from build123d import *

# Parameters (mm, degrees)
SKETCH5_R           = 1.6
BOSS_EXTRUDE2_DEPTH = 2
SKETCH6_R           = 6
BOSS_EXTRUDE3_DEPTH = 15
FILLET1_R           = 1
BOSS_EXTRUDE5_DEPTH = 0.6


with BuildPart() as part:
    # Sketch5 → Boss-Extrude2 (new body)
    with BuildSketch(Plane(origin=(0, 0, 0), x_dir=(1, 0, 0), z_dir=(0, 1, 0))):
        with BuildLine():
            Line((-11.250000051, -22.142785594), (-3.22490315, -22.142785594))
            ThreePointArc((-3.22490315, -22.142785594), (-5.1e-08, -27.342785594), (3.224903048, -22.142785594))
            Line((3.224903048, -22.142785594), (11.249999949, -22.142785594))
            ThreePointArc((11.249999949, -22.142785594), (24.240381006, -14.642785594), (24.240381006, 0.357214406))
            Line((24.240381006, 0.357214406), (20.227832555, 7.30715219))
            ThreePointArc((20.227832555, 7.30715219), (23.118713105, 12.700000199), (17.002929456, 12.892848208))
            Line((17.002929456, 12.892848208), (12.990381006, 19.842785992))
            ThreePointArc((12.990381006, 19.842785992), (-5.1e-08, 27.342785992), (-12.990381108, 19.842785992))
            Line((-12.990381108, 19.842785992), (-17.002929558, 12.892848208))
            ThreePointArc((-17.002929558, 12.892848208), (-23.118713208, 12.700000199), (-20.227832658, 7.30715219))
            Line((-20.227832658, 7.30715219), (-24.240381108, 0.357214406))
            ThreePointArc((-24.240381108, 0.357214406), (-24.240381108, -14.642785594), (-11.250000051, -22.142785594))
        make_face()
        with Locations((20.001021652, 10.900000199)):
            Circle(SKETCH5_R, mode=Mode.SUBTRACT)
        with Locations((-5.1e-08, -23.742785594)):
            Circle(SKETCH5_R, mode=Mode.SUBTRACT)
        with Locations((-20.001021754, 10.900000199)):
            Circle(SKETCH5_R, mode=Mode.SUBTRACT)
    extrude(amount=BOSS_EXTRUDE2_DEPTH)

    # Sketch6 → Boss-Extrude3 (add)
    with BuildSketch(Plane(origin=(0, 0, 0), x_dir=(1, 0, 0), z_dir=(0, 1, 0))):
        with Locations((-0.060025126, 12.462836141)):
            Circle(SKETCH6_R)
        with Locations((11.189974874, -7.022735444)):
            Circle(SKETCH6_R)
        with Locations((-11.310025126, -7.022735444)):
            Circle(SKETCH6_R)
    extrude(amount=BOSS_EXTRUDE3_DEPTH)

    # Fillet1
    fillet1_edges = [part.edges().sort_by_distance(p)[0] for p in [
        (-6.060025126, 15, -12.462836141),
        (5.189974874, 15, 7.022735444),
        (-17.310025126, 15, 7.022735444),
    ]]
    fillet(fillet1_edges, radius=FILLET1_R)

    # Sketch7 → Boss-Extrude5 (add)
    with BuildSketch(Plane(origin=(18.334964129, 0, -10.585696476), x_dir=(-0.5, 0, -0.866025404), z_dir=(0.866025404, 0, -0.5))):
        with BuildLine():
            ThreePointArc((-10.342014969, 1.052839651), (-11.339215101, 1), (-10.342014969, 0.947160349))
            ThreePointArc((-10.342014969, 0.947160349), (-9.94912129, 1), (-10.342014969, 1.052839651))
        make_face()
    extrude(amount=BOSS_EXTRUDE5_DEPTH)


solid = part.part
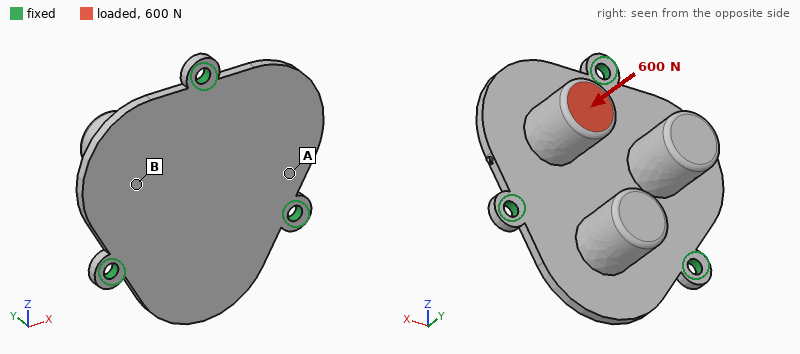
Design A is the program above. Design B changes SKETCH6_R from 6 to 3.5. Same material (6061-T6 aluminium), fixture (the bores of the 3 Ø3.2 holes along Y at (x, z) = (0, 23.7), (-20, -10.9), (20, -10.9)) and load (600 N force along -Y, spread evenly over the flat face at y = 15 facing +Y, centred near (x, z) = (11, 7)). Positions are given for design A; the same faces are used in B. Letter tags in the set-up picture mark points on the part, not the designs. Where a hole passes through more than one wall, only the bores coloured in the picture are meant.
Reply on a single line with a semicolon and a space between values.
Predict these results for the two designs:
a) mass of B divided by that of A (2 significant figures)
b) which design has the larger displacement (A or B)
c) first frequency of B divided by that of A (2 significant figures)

0.66; B; 1.1
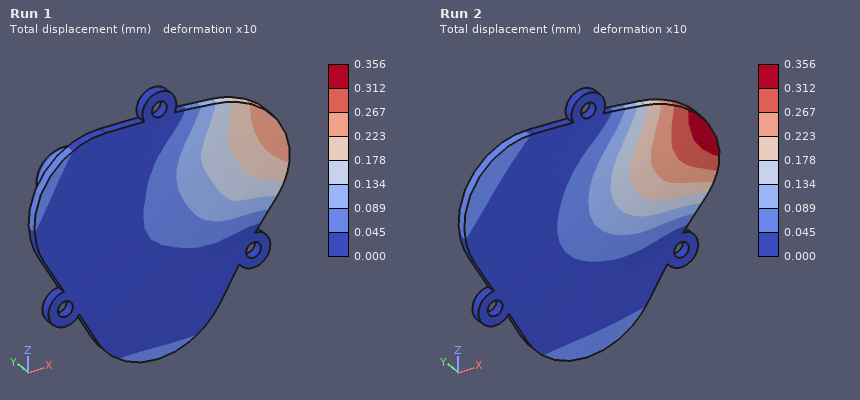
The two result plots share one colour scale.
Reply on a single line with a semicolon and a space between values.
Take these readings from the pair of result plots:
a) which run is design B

Run 2
